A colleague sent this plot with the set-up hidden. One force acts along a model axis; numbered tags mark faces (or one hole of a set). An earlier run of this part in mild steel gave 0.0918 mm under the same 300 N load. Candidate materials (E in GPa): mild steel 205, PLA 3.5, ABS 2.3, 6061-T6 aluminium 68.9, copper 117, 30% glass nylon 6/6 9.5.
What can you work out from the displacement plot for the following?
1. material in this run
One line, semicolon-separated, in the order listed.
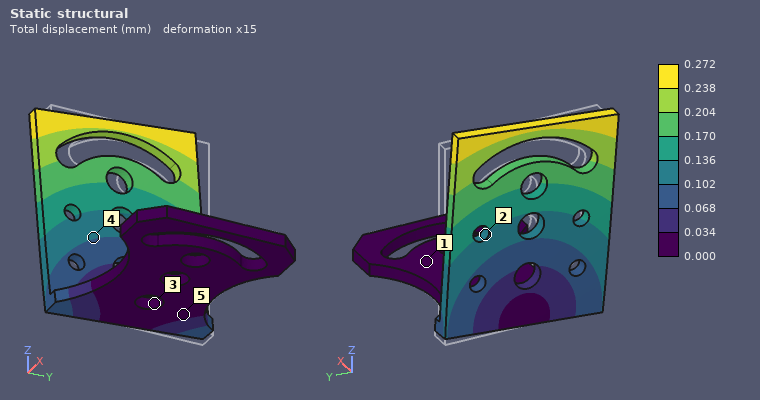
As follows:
6061-T6 aluminium
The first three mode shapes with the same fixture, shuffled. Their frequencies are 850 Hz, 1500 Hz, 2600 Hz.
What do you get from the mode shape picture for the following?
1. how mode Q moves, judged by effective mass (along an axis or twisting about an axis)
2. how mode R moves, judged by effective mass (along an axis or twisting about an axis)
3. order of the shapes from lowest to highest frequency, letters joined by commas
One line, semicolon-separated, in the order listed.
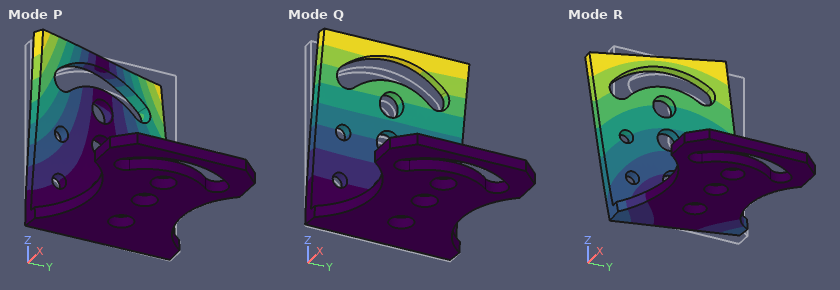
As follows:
along X; along Y; Q, R, P
